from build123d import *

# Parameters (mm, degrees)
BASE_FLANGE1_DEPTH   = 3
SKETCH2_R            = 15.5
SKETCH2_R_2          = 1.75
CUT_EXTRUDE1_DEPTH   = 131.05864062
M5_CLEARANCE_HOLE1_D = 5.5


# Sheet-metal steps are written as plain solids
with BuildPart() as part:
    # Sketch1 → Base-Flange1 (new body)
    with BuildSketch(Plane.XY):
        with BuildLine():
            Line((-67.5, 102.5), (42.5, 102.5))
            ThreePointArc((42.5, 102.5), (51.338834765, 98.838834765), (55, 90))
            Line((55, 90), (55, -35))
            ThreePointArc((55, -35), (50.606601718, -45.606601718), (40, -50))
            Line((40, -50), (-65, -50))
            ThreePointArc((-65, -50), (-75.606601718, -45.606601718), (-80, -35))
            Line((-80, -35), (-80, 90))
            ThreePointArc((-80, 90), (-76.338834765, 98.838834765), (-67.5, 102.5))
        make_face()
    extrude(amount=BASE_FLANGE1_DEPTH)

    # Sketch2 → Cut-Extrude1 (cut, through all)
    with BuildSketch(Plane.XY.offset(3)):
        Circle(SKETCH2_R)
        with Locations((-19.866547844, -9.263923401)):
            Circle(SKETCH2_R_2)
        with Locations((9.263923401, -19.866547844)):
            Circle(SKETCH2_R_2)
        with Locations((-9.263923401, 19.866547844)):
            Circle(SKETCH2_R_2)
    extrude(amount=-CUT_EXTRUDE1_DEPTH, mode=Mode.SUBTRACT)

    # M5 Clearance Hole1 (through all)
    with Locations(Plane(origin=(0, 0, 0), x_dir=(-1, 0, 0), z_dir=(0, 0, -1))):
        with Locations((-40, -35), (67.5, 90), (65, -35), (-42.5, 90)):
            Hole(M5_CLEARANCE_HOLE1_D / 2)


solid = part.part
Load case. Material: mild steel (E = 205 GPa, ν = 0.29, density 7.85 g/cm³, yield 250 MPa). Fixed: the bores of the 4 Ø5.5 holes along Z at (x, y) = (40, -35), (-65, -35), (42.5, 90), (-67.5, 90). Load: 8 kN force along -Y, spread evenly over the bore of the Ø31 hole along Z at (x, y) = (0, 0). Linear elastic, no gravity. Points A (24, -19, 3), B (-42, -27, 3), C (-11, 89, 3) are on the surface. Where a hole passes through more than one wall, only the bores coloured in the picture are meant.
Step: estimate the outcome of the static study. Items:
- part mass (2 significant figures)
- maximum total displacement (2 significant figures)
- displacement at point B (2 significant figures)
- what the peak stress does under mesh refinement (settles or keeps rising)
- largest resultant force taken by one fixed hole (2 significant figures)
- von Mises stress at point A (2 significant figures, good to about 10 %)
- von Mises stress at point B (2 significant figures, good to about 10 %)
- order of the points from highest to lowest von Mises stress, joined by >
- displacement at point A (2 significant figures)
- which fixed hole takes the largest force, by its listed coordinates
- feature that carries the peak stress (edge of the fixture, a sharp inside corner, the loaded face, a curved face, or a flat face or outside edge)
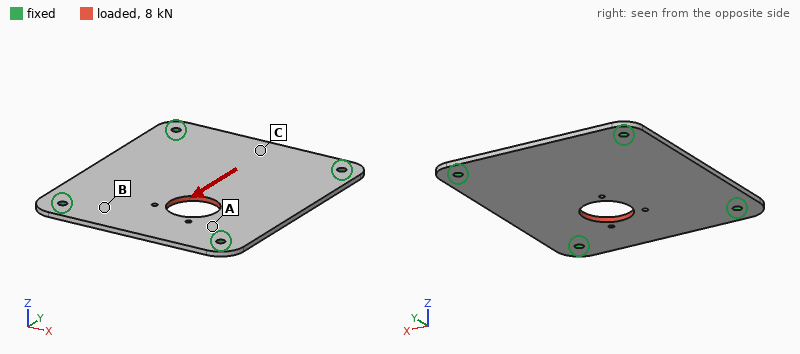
460 g
13 µm
5.5 µm
keeps rising
2.9 kN
29 MPa
18 MPa
A > B > C
6.3 µm
(40, -35)
edge of the fixture
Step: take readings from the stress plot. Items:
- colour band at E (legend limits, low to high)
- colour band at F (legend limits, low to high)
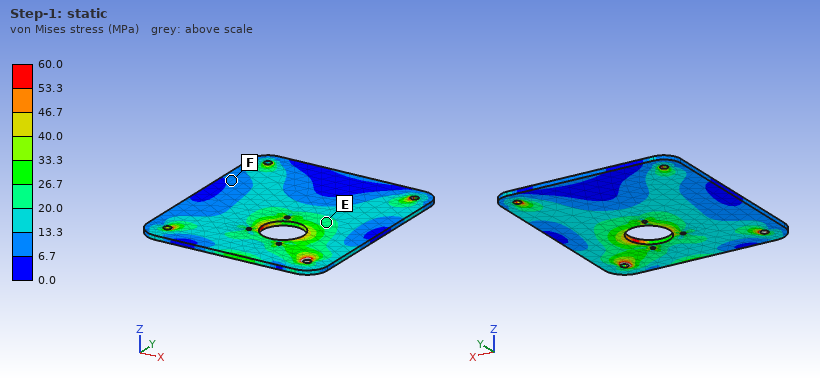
20.0 to 26.7 MPa
6.7 to 13.3 MPa
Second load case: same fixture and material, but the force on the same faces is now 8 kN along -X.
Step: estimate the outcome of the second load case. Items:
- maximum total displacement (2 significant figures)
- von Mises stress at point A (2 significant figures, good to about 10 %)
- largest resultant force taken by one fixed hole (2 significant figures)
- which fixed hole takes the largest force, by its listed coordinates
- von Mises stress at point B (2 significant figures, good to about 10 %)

13 µm
31 MPa
3.0 kN
(40, -35)
25 MPa
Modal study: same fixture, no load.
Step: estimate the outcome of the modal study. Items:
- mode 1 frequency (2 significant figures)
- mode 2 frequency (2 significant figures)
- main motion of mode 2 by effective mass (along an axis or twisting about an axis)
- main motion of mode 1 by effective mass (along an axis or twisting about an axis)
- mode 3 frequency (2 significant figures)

760 Hz
1200 Hz
twisting about Y
along Z
1400 Hz
